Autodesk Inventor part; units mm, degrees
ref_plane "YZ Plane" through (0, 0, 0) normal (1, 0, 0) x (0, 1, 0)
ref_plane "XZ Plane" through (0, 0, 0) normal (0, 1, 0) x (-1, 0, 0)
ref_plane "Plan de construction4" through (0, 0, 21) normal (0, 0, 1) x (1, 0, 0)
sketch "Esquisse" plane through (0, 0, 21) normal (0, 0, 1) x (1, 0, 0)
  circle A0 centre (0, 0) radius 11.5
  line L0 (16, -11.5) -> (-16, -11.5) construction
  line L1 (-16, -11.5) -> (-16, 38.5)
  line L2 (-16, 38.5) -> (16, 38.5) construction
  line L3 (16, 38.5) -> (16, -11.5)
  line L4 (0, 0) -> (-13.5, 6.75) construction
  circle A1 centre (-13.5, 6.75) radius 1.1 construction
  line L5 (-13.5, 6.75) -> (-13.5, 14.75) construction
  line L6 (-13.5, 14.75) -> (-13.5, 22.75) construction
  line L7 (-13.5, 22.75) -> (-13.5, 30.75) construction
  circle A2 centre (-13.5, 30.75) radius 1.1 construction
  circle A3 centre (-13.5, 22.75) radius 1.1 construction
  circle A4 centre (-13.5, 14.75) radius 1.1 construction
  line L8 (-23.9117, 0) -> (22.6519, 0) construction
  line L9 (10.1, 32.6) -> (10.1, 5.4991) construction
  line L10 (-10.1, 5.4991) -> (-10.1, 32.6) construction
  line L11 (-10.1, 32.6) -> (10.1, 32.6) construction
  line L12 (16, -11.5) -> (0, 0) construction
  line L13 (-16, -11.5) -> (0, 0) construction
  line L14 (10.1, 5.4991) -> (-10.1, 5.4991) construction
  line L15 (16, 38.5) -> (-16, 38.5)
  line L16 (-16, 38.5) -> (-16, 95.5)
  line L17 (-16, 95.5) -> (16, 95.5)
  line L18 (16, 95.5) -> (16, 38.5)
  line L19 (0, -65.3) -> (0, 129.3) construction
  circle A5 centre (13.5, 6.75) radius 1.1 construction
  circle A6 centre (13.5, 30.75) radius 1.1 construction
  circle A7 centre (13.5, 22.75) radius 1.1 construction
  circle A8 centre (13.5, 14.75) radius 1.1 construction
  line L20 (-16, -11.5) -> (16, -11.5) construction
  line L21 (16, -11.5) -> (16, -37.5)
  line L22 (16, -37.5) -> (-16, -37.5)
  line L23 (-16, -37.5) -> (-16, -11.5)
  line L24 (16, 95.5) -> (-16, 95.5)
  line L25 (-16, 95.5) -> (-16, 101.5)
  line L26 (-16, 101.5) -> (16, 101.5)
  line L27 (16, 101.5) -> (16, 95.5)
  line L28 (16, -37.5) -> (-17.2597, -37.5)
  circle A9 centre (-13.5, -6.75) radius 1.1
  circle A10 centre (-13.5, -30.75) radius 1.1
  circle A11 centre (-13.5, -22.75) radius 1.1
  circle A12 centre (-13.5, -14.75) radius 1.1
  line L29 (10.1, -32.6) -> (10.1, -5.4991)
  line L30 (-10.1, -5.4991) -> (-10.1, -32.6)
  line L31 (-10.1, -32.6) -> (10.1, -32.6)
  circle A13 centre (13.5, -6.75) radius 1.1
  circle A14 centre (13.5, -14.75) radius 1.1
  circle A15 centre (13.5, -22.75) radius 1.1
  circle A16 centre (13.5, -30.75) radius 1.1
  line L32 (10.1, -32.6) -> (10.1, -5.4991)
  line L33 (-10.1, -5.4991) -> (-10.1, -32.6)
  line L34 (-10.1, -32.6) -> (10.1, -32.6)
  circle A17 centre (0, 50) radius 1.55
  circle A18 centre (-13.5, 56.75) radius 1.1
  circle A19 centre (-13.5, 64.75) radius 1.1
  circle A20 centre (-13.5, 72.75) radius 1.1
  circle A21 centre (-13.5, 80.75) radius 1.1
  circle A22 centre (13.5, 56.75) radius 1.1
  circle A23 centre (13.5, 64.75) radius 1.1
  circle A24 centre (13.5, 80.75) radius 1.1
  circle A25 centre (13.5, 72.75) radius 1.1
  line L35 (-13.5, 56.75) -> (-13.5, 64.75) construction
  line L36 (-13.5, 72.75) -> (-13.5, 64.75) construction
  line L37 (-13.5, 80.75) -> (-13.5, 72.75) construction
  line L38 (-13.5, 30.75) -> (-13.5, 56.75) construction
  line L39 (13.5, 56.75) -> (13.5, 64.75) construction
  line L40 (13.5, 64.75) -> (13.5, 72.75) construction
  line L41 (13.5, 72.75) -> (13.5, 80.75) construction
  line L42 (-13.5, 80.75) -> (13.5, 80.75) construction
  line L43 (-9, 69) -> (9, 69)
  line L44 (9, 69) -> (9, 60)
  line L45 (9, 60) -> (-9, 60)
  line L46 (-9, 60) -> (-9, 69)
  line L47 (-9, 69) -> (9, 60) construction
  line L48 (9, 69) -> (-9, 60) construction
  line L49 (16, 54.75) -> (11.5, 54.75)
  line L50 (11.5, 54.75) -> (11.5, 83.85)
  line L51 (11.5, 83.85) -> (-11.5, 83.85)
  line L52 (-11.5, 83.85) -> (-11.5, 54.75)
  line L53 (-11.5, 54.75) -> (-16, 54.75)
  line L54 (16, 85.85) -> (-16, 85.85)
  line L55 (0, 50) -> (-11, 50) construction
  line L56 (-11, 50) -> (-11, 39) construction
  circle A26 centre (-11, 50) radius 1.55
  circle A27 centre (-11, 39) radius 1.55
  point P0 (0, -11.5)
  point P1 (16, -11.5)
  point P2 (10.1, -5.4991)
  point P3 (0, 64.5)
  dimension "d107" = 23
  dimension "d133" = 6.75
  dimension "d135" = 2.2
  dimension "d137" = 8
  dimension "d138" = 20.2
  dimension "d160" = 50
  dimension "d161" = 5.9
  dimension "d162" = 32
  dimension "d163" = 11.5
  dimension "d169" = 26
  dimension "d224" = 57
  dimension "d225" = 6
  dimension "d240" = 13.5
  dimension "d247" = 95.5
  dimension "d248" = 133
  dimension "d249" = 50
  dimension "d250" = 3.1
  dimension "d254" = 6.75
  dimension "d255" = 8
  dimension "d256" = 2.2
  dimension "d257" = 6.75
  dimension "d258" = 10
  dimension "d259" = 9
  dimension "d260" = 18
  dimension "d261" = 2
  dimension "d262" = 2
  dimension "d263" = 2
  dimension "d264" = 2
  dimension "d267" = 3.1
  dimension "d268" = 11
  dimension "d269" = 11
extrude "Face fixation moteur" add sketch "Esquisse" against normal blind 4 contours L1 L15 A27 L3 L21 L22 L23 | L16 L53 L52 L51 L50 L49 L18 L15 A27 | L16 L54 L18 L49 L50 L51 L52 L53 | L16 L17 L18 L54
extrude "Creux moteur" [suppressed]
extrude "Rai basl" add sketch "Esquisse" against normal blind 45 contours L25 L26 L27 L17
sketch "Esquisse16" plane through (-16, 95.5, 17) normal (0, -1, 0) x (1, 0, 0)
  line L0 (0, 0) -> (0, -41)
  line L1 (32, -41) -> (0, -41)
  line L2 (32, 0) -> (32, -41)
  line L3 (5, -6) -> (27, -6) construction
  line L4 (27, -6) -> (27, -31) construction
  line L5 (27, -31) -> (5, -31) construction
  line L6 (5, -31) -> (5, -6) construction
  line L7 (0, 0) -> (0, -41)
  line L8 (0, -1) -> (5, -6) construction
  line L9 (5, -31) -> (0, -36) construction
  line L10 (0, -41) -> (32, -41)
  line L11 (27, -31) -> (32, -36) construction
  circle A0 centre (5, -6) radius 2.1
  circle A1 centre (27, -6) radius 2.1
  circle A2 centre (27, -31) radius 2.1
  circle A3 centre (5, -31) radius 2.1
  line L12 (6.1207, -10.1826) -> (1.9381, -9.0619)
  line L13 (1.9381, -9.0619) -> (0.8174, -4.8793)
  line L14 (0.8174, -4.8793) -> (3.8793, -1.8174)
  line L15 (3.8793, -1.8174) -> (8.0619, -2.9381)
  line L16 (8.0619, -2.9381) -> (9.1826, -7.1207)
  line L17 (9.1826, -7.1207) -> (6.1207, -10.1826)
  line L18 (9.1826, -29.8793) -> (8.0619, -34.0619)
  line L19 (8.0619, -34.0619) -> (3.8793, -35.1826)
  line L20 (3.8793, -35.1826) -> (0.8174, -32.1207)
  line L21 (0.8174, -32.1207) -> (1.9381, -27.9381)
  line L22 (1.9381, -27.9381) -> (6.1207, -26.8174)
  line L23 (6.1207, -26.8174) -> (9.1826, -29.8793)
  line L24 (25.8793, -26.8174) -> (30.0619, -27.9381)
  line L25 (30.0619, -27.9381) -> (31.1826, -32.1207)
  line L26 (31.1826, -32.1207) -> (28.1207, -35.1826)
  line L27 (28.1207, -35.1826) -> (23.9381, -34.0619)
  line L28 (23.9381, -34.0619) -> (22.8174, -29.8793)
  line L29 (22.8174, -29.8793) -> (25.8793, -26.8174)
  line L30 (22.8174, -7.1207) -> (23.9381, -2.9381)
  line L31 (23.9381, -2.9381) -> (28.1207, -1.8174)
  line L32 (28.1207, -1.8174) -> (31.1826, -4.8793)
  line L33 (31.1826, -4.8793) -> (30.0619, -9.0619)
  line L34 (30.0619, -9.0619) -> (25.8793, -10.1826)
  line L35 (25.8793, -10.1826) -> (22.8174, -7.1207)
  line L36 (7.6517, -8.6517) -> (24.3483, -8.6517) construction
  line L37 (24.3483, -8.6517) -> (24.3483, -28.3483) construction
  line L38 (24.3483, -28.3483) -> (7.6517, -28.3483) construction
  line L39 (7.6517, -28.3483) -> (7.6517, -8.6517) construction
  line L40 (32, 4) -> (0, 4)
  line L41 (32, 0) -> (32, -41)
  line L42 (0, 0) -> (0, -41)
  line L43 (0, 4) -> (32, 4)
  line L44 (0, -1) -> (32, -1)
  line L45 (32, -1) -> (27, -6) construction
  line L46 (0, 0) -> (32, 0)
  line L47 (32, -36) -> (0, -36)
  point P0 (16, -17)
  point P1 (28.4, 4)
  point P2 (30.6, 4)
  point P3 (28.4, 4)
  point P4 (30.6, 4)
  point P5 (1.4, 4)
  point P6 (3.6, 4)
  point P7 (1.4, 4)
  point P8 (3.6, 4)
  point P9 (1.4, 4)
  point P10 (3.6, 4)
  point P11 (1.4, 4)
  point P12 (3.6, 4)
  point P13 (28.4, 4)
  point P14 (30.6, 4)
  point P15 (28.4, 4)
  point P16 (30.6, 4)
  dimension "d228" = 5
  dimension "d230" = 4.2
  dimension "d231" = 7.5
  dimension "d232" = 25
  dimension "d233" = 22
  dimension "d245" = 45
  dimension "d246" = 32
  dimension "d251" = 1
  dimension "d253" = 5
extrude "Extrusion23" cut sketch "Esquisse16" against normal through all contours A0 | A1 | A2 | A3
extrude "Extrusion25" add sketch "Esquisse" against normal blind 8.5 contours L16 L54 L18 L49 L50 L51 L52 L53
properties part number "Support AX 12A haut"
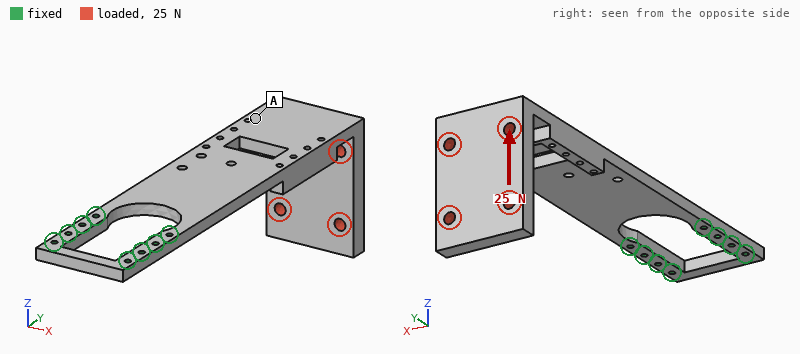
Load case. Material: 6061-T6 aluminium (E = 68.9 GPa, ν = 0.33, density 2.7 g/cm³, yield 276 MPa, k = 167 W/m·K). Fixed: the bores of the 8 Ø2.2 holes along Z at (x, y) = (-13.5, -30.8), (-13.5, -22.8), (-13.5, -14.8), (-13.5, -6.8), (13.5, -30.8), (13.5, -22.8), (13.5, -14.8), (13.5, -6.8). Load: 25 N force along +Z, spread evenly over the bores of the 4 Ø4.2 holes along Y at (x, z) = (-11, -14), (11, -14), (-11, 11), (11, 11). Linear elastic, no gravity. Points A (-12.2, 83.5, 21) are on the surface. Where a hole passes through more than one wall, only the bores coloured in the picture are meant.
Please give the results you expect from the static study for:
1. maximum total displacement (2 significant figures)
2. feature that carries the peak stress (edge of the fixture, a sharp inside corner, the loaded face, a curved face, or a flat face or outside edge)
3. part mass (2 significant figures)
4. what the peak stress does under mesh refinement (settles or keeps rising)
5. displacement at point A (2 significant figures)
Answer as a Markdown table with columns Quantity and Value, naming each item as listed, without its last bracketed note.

| Quantity | Value |
|---|---|
| maximum total displacement | 1.8 mm |
| feature that carries the peak stress | edge of the fixture |
| part mass | 60 g |
| what the peak stress does under mesh refinement | keeps rising |
| displacement at point A | 1.3 mm |
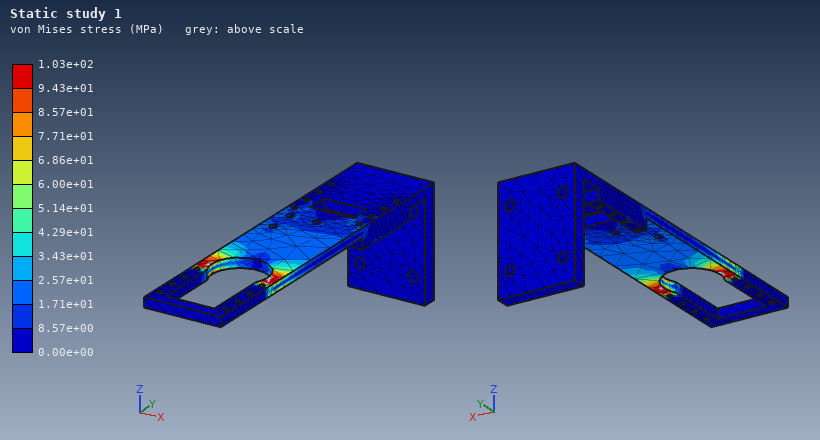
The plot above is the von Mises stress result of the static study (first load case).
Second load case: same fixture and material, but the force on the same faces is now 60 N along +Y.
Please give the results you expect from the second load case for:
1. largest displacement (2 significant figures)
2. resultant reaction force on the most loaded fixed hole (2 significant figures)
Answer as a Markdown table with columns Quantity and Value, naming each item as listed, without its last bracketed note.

| Quantity | Value |
|---|---|
| largest displacement | 1.1 mm |
| resultant reaction force on the most loaded fixed hole | 30 N |
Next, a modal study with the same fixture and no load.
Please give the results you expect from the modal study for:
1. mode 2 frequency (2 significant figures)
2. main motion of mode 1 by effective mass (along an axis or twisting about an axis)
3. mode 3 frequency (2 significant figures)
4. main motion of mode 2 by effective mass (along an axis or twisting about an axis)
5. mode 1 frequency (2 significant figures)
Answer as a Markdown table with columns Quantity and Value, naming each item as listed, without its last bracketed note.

| Quantity | Value |
|---|---|
| mode 2 frequency | 470 Hz |
| main motion of mode 1 by effective mass | along Z |
| mode 3 frequency | 810 Hz |
| main motion of mode 2 by effective mass | along X |
| mode 1 frequency | 110 Hz |
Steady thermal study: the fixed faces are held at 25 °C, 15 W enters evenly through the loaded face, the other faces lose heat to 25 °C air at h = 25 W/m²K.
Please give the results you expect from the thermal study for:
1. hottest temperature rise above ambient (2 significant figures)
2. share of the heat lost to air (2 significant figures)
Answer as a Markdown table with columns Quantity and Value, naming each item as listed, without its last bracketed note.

| Quantity | Value |
|---|---|
| hottest temperature rise above ambient | 54 K |
| share of the heat lost to air | 66 % |
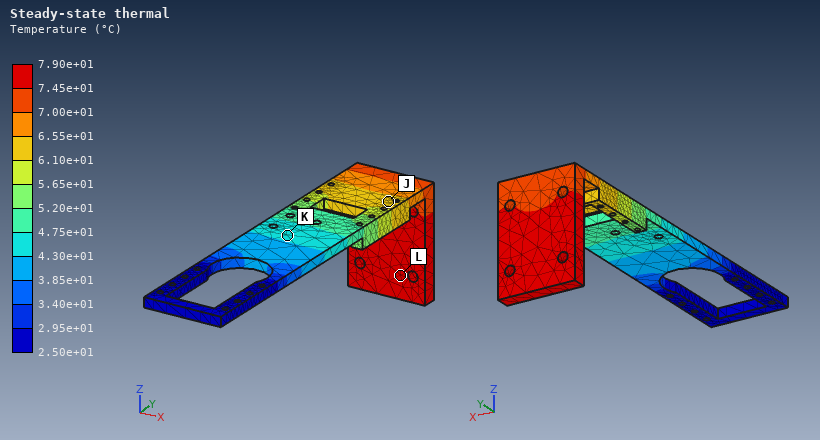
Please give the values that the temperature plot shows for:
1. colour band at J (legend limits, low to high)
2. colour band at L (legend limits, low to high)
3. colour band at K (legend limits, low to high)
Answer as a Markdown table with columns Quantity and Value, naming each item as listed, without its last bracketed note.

| Quantity | Value |
|---|---|
| colour band at J | 6.10e+01 to 6.55e+01 °C |
| colour band at L | 7.45e+01 to 7.90e+01 °C |
| colour band at K | 4.30e+01 to 4.75e+01 °C |
